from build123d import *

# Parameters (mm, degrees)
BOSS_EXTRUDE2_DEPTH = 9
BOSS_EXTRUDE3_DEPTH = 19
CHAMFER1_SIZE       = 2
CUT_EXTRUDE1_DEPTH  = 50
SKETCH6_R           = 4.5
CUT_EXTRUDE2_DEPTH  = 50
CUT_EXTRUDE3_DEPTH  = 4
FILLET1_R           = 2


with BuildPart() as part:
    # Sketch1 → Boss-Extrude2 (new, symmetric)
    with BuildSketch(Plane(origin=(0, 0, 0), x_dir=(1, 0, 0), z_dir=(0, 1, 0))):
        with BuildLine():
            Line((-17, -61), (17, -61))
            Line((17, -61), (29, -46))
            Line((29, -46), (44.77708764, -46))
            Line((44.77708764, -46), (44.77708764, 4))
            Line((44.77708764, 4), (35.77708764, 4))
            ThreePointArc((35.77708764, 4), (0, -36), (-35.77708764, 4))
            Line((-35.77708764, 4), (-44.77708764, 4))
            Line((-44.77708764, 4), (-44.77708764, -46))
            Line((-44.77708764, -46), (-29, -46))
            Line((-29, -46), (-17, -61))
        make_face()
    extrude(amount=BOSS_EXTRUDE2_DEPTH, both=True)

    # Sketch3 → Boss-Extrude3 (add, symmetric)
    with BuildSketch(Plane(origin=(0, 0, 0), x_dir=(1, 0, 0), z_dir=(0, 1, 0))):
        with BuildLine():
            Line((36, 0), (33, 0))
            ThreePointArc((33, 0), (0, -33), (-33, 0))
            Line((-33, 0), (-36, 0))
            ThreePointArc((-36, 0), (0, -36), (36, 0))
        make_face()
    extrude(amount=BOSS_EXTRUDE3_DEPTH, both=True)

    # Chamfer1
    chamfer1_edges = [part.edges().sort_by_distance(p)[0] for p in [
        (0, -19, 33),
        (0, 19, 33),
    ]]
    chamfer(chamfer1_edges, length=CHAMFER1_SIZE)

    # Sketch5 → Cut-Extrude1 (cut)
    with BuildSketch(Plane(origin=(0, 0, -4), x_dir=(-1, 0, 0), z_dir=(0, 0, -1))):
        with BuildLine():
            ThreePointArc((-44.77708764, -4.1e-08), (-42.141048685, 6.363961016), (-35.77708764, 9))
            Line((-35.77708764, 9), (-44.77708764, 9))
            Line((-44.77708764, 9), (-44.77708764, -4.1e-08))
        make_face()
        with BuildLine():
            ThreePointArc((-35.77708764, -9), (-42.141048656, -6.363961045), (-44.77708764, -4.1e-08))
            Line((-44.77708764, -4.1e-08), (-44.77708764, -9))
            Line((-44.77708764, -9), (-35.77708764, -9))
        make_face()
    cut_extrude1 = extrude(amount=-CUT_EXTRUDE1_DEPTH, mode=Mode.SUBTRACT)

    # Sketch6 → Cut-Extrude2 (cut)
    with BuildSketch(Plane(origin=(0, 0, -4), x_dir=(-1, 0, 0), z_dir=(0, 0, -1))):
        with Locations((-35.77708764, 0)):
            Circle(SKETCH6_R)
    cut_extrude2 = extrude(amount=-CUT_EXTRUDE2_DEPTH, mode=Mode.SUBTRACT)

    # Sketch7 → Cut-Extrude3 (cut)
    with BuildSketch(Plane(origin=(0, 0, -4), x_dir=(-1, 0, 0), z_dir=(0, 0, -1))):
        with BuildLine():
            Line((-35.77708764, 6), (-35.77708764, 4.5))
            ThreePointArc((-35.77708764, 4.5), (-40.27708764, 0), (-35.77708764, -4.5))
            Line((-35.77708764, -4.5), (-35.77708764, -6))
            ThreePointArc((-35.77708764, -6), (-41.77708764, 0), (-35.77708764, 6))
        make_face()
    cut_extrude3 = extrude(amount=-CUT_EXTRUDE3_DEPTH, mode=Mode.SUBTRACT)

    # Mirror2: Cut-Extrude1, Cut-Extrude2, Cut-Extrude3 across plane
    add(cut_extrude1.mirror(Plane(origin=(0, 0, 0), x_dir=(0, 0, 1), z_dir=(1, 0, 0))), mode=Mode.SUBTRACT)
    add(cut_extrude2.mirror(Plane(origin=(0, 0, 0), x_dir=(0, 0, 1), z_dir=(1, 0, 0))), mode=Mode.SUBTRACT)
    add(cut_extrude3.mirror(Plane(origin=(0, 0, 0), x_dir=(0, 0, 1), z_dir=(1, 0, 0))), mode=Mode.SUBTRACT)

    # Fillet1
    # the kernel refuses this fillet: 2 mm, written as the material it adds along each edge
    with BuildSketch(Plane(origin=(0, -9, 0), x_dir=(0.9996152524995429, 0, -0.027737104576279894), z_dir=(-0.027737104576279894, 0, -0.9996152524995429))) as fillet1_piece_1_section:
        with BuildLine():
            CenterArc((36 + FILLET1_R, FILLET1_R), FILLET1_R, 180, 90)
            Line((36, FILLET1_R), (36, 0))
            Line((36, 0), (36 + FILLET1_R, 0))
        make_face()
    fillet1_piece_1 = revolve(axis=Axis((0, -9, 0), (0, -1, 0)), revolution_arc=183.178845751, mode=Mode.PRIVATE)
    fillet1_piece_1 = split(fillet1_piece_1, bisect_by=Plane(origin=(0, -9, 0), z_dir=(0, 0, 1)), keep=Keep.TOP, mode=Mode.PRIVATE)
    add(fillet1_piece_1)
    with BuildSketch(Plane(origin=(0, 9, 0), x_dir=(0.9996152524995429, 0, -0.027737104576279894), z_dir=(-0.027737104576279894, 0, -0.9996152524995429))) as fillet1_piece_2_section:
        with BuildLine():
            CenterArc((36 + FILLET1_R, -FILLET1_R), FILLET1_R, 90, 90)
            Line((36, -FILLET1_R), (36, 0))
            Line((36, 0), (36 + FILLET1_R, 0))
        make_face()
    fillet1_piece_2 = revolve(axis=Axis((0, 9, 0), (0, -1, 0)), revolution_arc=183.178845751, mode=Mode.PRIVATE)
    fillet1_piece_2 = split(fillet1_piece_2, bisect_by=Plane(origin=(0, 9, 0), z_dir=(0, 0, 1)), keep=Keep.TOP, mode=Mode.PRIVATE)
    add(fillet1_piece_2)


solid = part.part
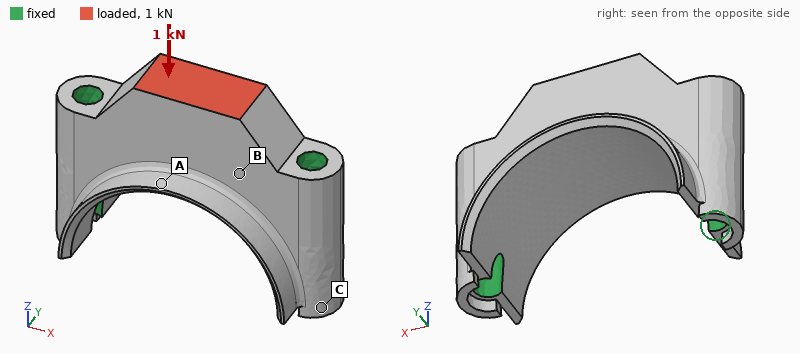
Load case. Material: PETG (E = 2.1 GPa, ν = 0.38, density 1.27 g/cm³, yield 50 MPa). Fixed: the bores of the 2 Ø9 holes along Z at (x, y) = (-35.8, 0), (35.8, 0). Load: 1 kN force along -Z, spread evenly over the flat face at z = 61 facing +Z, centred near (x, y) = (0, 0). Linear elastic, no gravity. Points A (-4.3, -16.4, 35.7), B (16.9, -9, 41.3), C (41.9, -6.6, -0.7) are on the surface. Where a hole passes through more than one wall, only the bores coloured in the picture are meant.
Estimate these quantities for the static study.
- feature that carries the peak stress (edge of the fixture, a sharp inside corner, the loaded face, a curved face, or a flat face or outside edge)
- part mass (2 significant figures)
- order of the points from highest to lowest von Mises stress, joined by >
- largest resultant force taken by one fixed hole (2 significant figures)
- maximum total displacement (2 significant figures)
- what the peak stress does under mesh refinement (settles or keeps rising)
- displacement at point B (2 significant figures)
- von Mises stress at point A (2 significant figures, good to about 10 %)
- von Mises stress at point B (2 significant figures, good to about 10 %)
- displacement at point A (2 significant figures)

edge of the fixture
68 g
B > A > C
610 N
49 µm
keeps rising
26 µm
0.77 MPa
1.8 MPa
35 µm
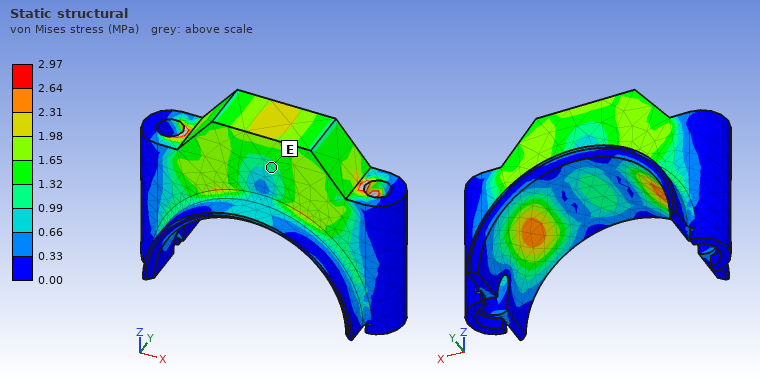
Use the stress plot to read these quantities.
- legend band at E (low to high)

0.99 to 1.32 MPa
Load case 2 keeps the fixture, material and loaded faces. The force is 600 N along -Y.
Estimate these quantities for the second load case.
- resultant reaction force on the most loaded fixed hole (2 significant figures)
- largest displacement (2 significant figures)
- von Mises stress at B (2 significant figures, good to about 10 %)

300 N
0.26 mm
4.9 MPa
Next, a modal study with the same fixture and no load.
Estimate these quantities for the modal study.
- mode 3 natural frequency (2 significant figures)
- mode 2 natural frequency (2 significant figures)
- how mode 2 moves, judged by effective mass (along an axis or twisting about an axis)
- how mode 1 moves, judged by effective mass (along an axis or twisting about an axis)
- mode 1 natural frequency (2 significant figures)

5100 Hz
4700 Hz
along Z
along Y
2600 Hz
